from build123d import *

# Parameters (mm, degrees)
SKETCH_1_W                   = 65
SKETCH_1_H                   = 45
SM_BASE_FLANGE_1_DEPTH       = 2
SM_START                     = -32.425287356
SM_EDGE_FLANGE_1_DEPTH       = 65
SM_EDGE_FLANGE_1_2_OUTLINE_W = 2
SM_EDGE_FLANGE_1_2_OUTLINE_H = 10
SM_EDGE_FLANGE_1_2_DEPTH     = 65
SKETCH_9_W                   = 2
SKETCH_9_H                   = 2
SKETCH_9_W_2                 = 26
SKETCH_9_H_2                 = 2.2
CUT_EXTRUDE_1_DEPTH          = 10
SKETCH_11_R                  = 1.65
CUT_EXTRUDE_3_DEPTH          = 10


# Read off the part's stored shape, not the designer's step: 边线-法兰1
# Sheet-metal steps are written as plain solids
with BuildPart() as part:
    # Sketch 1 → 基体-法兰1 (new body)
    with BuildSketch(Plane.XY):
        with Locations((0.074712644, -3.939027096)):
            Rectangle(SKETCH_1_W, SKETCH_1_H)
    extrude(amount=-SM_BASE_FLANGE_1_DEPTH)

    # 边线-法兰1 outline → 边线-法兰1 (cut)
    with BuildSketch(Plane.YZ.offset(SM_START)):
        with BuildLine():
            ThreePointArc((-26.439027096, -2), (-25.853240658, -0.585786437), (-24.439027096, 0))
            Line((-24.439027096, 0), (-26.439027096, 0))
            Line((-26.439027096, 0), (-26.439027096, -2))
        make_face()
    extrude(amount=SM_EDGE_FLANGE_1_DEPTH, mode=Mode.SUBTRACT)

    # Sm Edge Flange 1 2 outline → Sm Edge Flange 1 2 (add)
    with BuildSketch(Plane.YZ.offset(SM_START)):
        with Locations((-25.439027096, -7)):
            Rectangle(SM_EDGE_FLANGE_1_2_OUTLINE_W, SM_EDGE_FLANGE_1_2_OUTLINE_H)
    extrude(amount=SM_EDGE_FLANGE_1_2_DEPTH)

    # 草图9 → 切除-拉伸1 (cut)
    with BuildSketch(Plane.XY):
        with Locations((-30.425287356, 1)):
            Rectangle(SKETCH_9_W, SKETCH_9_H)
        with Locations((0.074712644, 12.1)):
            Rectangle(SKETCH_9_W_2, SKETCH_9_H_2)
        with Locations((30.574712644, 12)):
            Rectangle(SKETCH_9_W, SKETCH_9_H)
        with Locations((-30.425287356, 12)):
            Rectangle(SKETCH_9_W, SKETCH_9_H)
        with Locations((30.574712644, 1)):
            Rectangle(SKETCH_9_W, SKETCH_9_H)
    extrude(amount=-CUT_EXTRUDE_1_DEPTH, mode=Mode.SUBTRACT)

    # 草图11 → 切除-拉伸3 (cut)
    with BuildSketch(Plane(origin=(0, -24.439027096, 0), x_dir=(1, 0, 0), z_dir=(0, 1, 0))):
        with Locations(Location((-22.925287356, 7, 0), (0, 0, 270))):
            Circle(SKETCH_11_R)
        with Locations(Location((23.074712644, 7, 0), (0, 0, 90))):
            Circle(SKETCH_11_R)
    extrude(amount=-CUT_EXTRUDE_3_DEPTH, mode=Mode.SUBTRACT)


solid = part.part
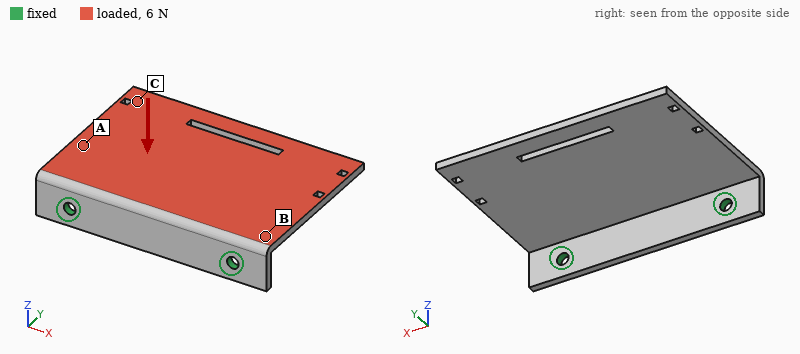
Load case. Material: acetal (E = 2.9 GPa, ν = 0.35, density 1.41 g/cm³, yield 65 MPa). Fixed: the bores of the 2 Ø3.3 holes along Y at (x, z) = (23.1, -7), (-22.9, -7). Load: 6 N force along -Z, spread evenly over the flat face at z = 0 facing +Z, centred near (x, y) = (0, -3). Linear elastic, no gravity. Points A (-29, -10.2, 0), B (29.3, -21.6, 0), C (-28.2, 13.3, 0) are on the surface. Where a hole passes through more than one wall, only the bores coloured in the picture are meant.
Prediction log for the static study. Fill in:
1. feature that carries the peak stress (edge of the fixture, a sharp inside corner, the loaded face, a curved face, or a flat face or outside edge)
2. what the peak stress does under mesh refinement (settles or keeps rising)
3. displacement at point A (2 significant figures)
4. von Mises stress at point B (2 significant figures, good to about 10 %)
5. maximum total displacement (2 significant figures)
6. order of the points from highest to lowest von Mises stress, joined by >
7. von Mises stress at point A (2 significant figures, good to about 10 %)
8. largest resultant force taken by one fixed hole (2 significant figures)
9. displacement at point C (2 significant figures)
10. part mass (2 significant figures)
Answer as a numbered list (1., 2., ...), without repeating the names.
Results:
1. edge of the fixture
2. keeps rising
3. 0.22 mm
4. 2.7 MPa
5. 0.90 mm
6. B > A > C
7. 1.5 MPa
8. 3.2 N
9. 0.75 mm
10. 9.7 g
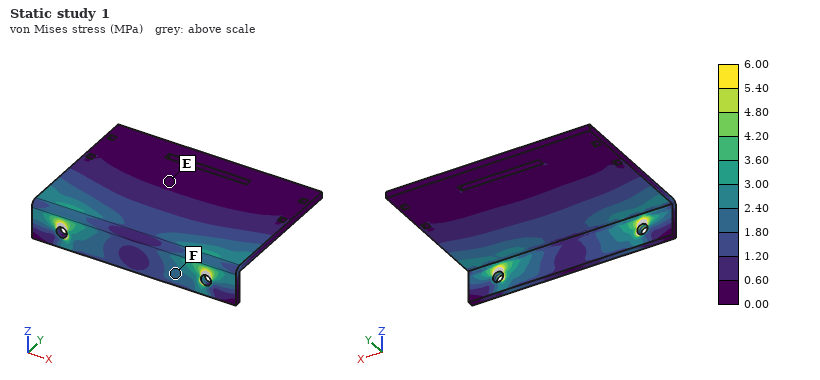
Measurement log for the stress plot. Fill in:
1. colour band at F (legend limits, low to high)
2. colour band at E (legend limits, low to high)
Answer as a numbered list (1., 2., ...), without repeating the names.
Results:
1. 1.80 to 2.40 MPa
2. 0.00 to 0.60 MPa
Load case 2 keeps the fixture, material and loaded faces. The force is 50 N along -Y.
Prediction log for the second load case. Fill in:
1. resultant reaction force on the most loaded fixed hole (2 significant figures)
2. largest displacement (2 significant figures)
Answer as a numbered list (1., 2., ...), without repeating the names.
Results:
1. 25 N
2. 0.88 mm
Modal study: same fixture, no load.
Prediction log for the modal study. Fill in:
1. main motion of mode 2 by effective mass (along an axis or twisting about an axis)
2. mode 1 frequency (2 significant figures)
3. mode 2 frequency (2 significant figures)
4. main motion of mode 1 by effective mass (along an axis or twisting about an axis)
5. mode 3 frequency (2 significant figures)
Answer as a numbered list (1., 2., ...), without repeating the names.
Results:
1. twisting about Y
2. 190 Hz
3. 400 Hz
4. along Z
5. 990 Hz
